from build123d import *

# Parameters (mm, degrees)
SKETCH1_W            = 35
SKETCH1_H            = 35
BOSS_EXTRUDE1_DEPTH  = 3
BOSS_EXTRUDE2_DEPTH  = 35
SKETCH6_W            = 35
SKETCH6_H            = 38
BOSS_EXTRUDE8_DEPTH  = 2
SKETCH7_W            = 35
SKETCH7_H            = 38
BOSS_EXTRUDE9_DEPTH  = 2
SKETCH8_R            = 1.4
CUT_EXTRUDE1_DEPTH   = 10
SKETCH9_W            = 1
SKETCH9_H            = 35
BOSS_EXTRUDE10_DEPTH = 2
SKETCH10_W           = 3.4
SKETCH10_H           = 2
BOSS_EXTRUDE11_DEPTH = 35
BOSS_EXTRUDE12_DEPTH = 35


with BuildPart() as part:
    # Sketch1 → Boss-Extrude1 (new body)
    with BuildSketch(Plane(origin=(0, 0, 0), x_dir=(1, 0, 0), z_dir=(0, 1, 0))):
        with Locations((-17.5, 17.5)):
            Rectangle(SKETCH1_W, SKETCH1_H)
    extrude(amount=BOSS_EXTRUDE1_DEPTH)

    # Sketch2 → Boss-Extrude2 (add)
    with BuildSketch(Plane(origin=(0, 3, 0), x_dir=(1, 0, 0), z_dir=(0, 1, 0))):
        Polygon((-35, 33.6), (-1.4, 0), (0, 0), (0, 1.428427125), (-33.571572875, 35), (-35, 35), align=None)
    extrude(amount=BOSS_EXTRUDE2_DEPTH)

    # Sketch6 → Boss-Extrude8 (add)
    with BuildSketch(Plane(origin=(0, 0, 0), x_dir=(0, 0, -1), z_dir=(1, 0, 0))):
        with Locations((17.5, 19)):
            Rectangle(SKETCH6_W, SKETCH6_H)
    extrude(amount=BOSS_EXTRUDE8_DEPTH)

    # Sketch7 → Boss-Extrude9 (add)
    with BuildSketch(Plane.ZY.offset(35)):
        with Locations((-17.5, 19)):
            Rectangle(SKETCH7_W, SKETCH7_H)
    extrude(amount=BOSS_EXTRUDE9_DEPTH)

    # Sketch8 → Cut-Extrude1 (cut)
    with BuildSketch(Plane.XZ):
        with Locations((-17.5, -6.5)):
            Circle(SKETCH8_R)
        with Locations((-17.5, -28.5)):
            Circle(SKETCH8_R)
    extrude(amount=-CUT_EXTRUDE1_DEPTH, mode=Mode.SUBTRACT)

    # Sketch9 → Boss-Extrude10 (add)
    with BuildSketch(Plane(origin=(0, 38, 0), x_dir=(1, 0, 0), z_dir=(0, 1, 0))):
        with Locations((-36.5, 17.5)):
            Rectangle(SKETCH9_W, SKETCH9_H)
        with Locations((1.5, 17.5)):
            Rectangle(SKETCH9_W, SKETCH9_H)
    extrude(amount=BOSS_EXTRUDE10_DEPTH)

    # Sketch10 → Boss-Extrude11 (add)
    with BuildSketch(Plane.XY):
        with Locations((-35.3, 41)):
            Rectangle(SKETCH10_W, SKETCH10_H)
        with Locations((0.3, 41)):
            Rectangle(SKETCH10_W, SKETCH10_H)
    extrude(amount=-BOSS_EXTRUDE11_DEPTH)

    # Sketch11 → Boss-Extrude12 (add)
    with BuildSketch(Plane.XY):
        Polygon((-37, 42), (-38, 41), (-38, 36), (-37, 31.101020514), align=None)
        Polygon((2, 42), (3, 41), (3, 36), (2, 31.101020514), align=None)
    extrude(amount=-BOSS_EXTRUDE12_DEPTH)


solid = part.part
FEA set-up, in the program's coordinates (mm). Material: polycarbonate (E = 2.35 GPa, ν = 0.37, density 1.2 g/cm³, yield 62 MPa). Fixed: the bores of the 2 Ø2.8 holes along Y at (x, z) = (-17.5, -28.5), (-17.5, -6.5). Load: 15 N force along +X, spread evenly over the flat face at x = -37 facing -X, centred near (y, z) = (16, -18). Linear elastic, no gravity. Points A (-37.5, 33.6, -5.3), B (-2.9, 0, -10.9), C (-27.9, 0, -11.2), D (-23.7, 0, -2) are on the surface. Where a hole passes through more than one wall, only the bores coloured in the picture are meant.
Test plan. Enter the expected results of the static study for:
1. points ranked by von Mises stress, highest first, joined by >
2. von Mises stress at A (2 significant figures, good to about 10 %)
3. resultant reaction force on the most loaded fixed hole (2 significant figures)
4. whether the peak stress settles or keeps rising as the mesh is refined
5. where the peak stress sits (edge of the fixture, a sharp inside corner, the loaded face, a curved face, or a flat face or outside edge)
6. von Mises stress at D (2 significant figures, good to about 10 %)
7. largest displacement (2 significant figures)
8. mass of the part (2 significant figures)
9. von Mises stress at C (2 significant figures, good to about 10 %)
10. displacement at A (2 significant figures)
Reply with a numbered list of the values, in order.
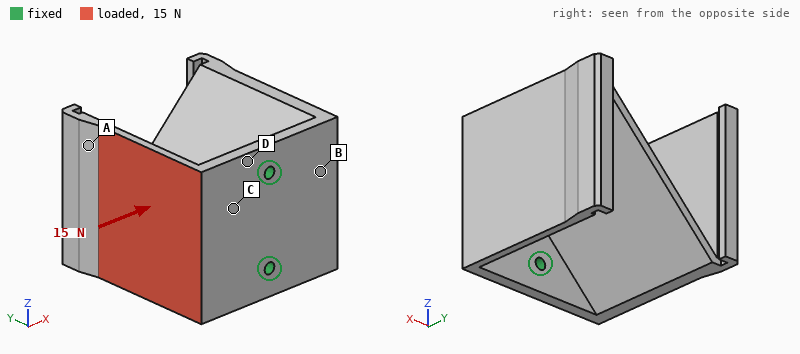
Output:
1. D > C > A > B
2. 0.80 MPa
3. 7.6 N
4. keeps rising
5. edge of the fixture
6. 2.6 MPa
7. 0.73 mm
8. 16 g
9. 1.8 MPa
10. 0.56 mm
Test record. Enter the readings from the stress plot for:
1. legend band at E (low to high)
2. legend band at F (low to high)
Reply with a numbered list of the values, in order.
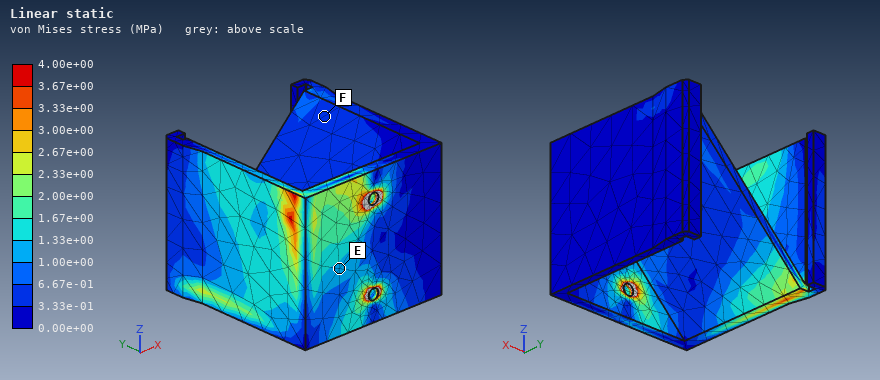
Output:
1. 1.00e+00 to 1.33e+00 MPa
2. 3.33e-01 to 6.67e-01 MPa
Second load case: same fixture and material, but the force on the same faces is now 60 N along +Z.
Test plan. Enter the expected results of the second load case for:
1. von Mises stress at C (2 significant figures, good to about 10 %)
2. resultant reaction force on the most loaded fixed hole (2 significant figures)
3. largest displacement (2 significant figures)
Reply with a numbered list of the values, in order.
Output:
1. 3.5 MPa
2. 70 N
3. 0.63 mm
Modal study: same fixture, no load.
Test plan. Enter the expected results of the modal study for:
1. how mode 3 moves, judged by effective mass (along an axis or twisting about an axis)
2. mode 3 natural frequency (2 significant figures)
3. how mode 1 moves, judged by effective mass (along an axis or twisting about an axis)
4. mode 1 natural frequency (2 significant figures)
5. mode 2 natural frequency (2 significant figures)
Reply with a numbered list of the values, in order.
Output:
1. along Z
2. 710 Hz
3. along X
4. 300 Hz
5. 420 Hz
